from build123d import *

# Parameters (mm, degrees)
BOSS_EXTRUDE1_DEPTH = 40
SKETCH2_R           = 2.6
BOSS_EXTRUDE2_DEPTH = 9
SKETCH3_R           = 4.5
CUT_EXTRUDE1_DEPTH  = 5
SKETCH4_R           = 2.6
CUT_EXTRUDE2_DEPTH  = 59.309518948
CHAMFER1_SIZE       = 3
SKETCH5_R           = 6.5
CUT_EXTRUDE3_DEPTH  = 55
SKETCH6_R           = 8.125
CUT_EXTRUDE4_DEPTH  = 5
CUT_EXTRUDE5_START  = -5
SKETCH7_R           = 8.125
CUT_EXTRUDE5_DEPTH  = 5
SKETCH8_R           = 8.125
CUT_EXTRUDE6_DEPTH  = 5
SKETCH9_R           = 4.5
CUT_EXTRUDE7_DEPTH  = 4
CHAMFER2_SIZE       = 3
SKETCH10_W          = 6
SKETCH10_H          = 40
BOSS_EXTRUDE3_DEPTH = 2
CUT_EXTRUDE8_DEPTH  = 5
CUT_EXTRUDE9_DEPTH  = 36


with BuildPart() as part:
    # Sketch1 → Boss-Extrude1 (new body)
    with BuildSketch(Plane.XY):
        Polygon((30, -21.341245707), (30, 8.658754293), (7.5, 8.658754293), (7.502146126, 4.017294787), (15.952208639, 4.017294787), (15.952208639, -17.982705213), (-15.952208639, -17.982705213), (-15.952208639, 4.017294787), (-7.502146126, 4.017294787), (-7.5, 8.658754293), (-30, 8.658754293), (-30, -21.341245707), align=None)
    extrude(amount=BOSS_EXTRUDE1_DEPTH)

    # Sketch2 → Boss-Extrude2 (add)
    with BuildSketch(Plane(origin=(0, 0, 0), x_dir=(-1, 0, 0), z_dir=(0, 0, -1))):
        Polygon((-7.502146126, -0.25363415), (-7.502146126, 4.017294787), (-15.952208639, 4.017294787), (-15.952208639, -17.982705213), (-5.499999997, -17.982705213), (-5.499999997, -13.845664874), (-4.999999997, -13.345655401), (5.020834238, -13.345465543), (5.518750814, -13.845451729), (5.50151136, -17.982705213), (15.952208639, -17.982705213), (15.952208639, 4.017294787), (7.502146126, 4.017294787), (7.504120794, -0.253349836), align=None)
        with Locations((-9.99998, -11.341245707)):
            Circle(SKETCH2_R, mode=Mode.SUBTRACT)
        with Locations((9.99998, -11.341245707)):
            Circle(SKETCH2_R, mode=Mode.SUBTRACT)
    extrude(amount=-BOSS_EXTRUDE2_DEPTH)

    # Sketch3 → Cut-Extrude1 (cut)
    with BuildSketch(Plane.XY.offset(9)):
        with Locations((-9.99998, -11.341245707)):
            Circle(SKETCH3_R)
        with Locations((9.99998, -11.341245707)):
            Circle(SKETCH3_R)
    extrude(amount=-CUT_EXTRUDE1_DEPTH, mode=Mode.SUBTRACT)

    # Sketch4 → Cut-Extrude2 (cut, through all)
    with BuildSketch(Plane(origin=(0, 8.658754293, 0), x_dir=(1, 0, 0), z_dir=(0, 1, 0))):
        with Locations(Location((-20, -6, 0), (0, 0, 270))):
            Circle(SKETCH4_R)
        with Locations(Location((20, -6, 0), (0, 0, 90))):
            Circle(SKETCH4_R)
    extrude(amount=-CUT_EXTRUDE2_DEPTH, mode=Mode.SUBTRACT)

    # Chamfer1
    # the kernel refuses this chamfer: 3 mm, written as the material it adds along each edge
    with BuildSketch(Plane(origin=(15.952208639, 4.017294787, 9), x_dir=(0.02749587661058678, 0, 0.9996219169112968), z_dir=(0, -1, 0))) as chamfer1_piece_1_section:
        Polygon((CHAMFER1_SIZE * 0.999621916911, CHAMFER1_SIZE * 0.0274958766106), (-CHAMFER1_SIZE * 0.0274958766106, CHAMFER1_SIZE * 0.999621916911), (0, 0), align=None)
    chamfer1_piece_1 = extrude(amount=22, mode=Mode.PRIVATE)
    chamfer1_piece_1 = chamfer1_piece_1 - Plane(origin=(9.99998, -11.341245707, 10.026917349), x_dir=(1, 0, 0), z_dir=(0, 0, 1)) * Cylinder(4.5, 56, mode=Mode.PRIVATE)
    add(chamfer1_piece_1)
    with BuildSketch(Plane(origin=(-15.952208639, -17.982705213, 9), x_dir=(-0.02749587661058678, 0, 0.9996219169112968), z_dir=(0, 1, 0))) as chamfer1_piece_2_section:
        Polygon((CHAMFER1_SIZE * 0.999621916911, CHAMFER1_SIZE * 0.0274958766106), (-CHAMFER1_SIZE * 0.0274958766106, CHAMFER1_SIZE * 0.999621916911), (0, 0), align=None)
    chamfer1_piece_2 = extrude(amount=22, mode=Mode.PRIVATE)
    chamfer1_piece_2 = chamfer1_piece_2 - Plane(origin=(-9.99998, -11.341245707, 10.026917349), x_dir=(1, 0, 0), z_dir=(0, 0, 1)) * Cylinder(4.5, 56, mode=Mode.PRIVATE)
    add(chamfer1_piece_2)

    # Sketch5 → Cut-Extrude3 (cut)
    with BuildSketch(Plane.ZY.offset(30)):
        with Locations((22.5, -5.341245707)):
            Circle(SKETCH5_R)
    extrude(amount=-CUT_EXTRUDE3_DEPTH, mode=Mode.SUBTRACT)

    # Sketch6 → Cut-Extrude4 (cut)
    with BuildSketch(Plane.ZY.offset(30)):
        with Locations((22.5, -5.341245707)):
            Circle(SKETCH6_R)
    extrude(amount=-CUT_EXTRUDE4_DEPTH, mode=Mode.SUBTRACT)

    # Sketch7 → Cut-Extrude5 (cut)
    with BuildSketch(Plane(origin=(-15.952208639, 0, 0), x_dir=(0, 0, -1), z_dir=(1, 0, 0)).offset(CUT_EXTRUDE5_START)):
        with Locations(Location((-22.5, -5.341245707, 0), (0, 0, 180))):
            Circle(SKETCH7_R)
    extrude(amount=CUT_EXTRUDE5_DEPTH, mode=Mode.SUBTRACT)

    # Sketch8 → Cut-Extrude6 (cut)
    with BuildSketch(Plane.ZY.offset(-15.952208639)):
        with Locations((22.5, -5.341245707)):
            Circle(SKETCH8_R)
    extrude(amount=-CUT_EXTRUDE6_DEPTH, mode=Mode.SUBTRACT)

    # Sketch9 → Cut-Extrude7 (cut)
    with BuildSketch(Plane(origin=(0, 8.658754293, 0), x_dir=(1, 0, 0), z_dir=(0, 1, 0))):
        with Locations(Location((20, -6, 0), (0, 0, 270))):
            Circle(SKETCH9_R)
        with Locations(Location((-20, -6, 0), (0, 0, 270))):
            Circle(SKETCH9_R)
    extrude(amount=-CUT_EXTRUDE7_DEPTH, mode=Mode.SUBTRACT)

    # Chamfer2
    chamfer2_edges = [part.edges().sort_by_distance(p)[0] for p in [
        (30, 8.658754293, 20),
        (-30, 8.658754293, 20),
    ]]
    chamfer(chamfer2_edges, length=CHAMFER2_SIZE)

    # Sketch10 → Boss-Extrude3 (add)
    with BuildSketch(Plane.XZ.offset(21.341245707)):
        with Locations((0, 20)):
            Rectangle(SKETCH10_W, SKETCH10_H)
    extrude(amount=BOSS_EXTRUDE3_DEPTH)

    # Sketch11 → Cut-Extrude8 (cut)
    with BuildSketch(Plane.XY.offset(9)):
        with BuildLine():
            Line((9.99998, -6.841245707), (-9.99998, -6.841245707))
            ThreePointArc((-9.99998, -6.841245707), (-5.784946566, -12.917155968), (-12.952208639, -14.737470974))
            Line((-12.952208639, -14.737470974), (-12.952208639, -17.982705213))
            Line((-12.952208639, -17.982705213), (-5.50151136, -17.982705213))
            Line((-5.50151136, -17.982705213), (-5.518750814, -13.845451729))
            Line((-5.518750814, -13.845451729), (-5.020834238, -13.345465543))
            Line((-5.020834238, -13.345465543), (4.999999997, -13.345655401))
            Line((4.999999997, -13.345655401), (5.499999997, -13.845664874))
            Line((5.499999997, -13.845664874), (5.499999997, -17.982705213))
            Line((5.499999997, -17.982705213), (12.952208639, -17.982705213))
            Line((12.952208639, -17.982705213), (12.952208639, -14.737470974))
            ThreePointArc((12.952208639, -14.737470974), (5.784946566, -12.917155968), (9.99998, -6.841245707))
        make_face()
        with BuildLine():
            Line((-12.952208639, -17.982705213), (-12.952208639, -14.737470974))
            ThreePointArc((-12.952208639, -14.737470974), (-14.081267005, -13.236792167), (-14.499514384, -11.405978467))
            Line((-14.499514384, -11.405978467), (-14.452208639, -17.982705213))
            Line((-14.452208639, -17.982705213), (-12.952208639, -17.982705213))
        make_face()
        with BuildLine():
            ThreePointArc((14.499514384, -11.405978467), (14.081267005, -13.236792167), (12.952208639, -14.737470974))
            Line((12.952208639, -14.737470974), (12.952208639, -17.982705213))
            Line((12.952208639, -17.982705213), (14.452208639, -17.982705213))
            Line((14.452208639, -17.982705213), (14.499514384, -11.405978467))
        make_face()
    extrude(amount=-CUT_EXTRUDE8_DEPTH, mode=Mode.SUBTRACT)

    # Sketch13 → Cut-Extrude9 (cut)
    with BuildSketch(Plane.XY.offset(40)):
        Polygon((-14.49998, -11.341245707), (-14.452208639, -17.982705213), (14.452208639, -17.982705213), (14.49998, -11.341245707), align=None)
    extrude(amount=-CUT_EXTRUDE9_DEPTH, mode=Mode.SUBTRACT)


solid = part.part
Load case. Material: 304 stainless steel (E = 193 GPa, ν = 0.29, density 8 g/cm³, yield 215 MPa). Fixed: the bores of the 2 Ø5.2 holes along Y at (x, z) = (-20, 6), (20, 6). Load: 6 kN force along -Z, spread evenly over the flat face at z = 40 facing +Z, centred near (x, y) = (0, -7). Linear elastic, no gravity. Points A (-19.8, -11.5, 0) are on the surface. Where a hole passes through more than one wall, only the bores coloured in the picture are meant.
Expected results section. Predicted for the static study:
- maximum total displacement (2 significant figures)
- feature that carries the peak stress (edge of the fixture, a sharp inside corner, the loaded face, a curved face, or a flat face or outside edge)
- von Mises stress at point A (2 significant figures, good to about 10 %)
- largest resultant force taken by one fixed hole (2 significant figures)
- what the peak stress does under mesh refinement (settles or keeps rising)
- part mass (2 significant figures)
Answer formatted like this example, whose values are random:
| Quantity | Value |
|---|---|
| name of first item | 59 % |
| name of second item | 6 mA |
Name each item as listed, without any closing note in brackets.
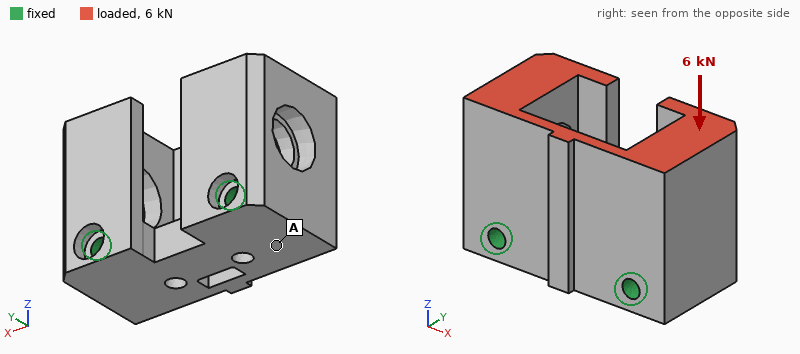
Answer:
| Quantity | Value |
|---|---|
| maximum total displacement | 2.9 µm |
| feature that carries the peak stress | edge of the fixture |
| von Mises stress at point A | 4.0 MPa |
| largest resultant force taken by one fixed hole | 3.0 kN |
| what the peak stress does under mesh refinement | keeps rising |
| part mass | 320 g |
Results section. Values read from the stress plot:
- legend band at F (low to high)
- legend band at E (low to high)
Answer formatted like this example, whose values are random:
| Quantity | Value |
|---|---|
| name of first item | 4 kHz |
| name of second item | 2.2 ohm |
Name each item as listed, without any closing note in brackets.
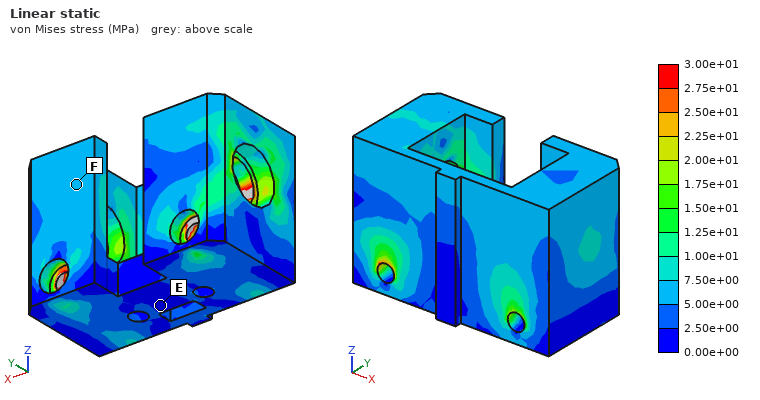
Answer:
| Quantity | Value |
|---|---|
| legend band at F | 5.00e+00 to 7.50e+00 MPa |
| legend band at E | 0.00e+00 to 2.50e+00 MPa |
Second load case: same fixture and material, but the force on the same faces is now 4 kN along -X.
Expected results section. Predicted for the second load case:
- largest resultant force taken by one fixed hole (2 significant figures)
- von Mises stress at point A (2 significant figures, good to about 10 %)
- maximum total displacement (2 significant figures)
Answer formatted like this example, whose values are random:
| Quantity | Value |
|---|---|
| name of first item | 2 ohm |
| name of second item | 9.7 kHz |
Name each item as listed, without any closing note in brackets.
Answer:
| Quantity | Value |
|---|---|
| largest resultant force taken by one fixed hole | 2.8 kN |
| von Mises stress at point A | 12 MPa |
| maximum total displacement | 20 µm |
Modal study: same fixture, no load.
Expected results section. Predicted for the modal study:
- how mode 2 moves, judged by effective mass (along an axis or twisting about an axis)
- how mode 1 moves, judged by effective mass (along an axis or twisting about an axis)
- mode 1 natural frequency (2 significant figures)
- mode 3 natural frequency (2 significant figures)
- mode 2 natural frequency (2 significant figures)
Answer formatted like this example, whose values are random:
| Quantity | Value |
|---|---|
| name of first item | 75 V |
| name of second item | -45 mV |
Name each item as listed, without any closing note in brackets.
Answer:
| Quantity | Value |
|---|---|
| how mode 2 moves, judged by effective mass | along X |
| how mode 1 moves, judged by effective mass | along Y |
| mode 1 natural frequency | 8100 Hz |
| mode 3 natural frequency | 9700 Hz |
| mode 2 natural frequency | 9200 Hz |
